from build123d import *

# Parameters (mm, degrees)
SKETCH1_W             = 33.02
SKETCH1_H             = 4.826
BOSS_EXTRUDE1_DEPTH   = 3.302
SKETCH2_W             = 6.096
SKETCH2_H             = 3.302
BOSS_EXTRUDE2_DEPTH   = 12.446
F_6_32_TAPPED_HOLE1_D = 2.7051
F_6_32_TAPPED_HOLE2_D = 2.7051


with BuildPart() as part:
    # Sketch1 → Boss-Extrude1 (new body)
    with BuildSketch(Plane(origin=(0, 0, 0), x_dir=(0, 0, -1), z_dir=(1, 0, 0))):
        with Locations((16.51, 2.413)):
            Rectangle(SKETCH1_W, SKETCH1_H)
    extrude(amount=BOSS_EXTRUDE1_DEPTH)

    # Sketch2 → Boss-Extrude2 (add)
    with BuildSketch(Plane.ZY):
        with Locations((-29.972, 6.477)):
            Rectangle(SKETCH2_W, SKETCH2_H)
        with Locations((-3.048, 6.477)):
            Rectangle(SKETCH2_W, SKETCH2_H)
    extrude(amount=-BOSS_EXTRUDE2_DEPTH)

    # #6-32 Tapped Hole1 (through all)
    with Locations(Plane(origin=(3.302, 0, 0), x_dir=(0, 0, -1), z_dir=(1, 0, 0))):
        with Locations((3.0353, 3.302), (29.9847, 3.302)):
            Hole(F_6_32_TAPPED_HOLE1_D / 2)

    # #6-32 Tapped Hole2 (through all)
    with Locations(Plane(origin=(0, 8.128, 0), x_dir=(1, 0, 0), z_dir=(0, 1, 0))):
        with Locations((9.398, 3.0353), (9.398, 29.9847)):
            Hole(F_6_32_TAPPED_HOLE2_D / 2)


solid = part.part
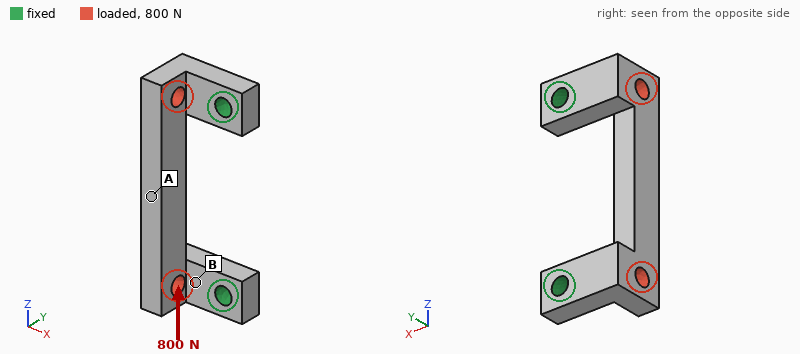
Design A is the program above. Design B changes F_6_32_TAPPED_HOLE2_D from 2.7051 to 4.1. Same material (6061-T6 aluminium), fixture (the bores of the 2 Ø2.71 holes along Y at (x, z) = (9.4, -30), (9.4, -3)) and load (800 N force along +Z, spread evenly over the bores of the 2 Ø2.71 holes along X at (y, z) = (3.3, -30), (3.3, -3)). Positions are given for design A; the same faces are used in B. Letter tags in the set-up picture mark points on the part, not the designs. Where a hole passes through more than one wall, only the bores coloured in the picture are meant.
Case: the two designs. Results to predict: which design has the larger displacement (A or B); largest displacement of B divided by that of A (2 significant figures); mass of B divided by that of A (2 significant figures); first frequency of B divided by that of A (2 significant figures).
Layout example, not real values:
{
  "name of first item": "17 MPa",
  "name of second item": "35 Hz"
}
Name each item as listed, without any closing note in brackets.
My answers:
{
  "which design has the larger displacement": "A",
  "largest displacement of B divided by that of A": "0.77",
  "mass of B divided by that of A": "0.95",
  "first frequency of B divided by that of A": "1.1"
}
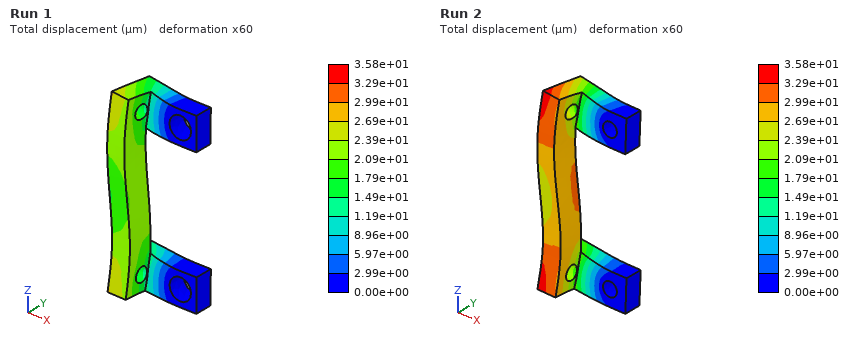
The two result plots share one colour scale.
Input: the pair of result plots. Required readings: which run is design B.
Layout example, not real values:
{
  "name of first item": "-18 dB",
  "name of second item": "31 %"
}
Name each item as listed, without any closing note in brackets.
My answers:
{
  "which run is design B": "Run 1"
}
